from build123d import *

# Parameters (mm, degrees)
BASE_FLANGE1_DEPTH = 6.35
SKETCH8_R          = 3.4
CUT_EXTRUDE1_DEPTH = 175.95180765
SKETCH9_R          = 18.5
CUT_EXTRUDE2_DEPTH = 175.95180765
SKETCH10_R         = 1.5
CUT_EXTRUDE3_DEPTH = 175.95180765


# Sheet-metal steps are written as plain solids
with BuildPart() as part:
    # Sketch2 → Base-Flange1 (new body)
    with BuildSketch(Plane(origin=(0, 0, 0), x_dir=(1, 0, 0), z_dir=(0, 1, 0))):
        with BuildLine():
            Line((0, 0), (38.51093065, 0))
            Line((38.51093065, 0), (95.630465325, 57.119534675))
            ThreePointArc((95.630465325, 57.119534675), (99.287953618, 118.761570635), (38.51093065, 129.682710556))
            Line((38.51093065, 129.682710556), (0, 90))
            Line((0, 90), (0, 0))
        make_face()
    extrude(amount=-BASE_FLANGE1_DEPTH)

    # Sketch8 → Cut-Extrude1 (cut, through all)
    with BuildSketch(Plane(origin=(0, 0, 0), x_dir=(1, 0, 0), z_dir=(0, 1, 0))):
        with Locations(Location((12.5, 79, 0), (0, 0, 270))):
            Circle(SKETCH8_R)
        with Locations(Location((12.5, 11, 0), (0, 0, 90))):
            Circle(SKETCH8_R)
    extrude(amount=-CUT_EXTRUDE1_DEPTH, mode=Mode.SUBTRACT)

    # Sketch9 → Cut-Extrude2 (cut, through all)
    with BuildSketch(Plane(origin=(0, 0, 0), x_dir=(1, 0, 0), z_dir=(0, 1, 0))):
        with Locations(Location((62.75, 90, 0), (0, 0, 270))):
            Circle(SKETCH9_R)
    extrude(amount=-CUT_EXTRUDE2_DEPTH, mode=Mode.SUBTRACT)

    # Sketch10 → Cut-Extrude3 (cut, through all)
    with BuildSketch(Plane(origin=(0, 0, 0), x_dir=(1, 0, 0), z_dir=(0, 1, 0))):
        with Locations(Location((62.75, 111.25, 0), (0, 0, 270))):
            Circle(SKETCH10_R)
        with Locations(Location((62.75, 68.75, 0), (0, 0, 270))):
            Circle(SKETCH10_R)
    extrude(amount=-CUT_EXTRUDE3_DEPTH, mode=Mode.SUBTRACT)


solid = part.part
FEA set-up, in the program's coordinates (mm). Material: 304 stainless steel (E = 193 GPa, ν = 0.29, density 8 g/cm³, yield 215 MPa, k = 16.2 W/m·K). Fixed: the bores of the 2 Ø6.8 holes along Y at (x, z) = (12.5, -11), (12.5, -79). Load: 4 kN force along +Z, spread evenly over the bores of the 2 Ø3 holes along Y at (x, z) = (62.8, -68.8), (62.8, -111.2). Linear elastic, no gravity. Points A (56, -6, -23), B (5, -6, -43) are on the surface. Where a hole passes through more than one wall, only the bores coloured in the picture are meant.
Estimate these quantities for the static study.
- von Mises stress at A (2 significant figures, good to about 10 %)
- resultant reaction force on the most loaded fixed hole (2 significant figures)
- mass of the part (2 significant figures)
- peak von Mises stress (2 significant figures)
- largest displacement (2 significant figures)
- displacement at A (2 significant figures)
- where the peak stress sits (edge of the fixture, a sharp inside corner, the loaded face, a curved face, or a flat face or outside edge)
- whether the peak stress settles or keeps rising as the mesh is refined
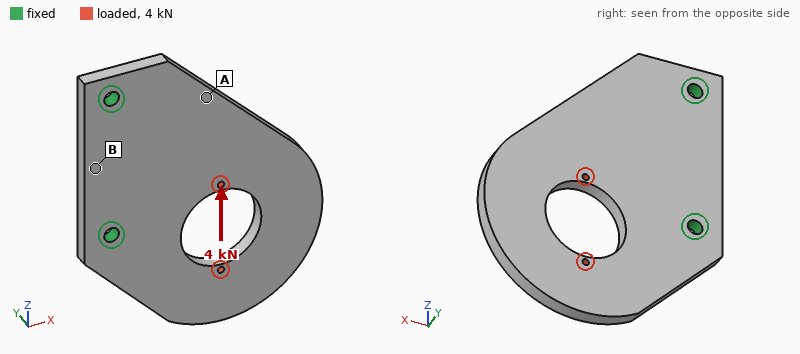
16 MPa
3.4 kN
490 g
110 MPa
20 µm
6.6 µm
a curved face
settles
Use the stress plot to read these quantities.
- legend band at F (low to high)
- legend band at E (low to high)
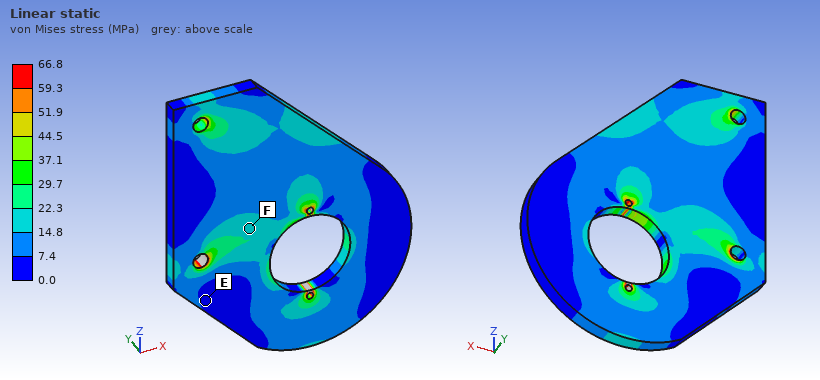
14.8 to 22.3 MPa
0.0 to 7.4 MPa
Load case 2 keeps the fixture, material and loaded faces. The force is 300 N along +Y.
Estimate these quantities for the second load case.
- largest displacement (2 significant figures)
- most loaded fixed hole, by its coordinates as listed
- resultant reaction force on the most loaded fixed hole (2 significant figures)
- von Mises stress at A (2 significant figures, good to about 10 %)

0.12 mm
(12.5, -79)
320 N
9.3 MPa
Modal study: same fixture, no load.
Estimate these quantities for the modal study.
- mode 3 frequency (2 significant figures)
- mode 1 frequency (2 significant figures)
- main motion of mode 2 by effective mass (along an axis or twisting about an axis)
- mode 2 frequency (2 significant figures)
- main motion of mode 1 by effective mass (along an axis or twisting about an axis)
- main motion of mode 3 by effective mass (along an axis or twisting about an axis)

2500 Hz
550 Hz
twisting about X
1200 Hz
along Y
along Y
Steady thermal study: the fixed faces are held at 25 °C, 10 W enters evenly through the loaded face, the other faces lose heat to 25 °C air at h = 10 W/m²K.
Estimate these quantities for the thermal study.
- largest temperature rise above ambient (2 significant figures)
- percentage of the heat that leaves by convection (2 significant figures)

72 K
53 %
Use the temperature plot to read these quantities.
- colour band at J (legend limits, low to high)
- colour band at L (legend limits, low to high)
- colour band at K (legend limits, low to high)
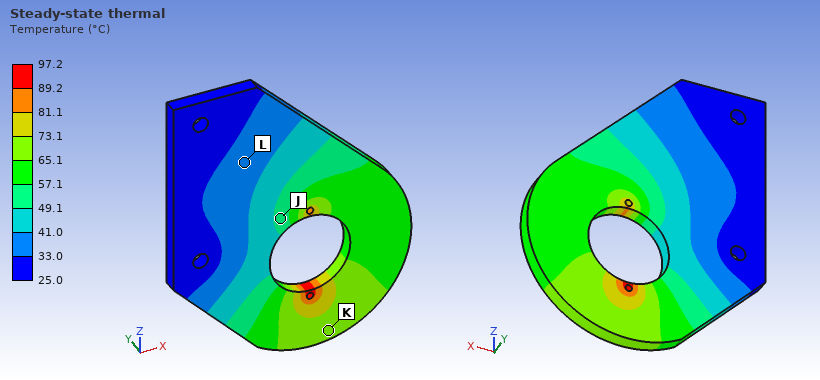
49.1 to 57.1 °C
33.0 to 41.0 °C
65.1 to 73.1 °C
